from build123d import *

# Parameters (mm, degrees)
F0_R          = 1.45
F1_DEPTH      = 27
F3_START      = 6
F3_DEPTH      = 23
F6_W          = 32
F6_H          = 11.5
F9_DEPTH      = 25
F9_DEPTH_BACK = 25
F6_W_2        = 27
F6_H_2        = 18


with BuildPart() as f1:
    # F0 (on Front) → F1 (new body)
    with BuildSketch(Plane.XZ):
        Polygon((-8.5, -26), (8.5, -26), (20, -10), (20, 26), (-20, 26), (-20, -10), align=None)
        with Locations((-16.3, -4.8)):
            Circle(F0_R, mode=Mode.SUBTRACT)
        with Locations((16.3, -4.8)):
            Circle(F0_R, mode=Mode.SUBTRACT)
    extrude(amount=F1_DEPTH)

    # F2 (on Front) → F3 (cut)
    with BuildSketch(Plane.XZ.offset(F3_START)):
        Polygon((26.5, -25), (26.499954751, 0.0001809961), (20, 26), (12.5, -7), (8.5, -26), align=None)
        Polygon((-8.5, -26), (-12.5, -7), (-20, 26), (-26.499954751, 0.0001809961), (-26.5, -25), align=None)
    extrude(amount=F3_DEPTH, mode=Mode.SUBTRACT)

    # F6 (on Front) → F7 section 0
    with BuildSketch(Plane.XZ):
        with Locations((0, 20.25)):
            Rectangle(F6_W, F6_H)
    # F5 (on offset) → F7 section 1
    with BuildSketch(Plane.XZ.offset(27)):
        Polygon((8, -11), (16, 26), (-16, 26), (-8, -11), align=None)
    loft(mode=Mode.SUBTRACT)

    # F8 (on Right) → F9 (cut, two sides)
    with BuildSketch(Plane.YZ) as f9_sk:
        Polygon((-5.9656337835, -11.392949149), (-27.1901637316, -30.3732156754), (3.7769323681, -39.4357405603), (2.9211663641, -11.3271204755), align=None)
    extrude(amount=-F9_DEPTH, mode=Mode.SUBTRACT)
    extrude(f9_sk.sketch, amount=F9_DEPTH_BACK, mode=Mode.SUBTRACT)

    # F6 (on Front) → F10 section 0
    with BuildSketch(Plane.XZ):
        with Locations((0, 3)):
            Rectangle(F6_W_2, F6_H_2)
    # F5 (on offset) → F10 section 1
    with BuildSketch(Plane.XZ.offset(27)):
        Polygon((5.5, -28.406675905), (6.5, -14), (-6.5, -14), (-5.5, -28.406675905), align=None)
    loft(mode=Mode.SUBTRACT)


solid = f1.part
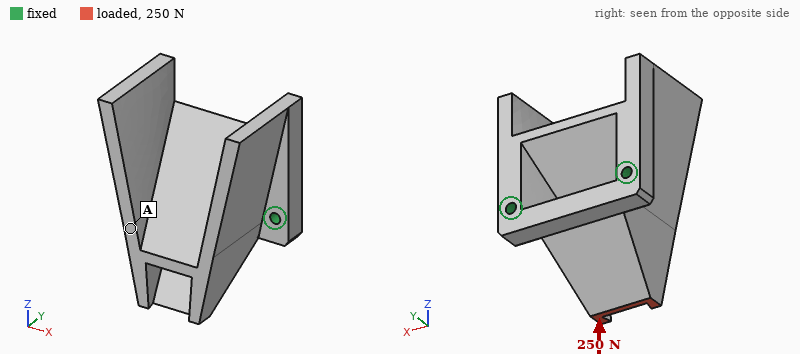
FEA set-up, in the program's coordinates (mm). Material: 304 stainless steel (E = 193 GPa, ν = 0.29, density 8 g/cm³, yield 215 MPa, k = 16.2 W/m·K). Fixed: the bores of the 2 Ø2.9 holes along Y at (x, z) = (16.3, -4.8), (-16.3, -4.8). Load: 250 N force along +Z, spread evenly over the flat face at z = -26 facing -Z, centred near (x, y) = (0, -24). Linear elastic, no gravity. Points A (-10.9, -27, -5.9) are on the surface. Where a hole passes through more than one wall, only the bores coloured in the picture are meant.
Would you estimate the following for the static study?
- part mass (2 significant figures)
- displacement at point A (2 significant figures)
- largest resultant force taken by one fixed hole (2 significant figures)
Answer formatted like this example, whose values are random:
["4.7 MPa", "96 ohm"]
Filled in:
["88 g", "8.8 µm", "130 N"]
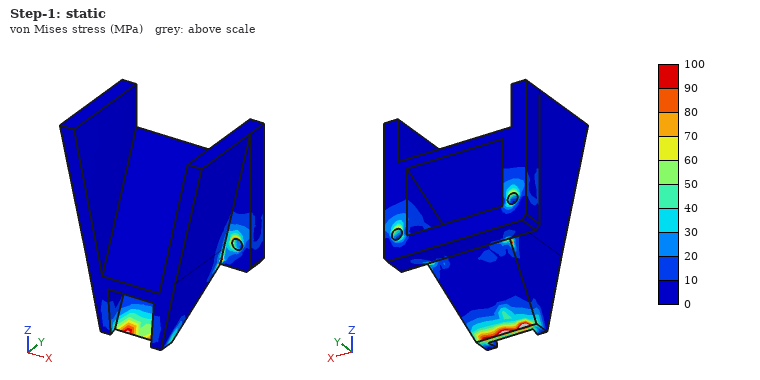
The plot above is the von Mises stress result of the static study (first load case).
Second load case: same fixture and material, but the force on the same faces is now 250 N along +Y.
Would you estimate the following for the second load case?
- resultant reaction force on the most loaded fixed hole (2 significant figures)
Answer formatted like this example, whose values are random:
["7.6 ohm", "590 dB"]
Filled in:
["130 N"]
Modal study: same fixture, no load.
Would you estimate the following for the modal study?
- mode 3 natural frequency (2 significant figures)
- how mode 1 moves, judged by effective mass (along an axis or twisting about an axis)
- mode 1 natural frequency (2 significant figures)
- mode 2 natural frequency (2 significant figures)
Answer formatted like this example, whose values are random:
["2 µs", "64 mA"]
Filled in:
["4400 Hz", "along X", "3100 Hz", "3300 Hz"]
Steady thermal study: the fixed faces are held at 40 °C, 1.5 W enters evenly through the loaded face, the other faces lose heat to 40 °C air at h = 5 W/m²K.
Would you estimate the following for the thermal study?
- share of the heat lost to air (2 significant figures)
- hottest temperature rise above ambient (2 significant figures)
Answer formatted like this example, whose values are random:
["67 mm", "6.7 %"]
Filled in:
["24 %", "45 K"]
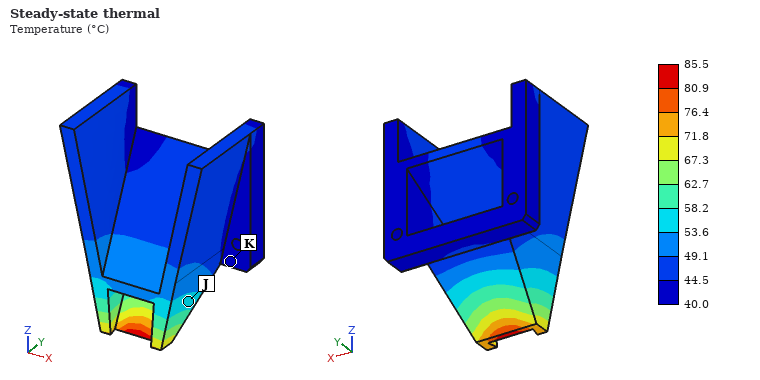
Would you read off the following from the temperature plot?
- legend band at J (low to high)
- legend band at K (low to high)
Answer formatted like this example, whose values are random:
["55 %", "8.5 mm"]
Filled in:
["53.6 to 58.2 °C", "40.0 to 44.5 °C"]
